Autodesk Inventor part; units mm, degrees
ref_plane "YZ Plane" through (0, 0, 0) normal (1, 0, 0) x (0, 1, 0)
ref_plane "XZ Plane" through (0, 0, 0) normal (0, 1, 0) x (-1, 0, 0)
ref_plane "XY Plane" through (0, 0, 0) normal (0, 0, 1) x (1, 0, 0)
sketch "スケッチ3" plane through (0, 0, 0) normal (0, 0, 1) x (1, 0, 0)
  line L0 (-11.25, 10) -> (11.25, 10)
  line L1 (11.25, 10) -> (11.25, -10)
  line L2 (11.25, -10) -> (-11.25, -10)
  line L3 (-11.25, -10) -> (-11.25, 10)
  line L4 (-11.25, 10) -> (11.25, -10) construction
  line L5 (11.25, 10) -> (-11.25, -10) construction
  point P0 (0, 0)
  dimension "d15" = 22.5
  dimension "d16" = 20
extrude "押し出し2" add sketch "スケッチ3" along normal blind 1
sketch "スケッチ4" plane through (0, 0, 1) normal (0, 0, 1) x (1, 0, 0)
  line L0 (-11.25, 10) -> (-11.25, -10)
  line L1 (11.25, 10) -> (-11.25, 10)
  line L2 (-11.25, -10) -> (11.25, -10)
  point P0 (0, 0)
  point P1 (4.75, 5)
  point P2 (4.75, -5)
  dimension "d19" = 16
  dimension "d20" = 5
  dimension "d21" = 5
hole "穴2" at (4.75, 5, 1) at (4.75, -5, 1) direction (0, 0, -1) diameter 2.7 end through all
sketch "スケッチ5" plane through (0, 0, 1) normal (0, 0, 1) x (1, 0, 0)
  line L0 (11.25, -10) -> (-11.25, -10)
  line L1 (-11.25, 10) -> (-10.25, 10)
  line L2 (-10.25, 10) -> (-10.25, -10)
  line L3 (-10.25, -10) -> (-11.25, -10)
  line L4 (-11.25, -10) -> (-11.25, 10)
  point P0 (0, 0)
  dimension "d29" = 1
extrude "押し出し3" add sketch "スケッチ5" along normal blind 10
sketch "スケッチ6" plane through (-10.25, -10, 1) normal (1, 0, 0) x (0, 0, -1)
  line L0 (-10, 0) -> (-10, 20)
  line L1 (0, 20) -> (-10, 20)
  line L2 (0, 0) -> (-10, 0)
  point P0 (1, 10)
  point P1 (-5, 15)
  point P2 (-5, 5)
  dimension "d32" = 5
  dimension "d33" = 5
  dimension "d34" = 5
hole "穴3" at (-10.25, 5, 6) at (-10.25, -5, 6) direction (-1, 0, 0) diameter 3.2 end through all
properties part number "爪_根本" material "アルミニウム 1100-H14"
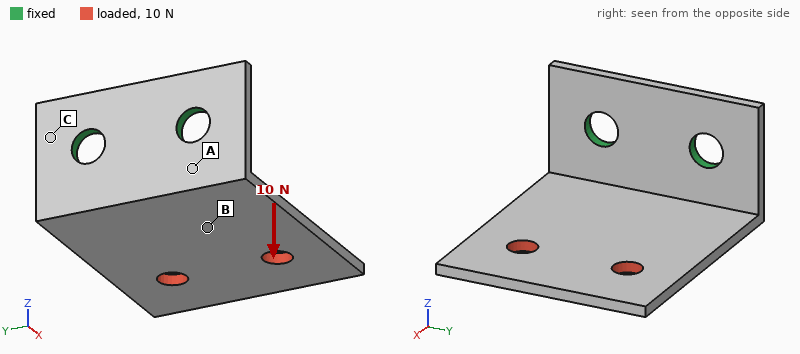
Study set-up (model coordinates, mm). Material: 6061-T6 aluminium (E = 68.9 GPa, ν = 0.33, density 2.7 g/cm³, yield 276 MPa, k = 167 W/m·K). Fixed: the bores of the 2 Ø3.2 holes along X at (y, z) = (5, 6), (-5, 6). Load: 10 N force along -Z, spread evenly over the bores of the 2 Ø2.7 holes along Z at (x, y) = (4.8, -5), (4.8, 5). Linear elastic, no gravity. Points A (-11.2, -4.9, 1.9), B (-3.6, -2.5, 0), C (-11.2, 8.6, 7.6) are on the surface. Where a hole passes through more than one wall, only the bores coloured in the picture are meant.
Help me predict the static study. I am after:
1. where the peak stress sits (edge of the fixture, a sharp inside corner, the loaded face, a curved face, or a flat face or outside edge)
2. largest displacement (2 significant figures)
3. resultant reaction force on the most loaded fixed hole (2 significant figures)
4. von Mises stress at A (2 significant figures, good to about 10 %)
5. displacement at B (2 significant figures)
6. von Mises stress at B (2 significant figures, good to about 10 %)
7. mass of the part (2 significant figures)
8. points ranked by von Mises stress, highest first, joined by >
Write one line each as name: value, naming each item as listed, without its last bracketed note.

where the peak stress sits: a flat face or outside edge
largest displacement: 0.28 mm
resultant reaction force on the most loaded fixed hole: 5.4 N
von Mises stress at A: 42 MPa
displacement at B: 0.068 mm
von Mises stress at B: 22 MPa
mass of the part: 1.7 g
points ranked by von Mises stress, highest first, joined by >: A > B > C
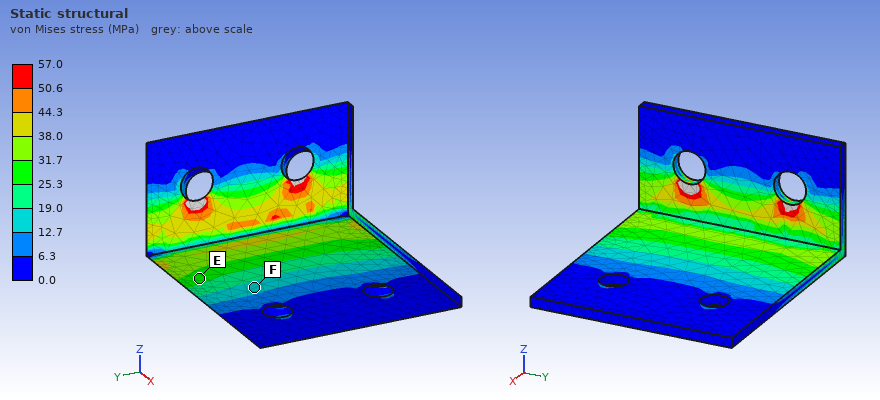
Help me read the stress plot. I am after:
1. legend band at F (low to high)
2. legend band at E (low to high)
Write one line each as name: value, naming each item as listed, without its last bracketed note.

legend band at F: 12.7 to 19.0 MPa
legend band at E: 25.3 to 31.7 MPa
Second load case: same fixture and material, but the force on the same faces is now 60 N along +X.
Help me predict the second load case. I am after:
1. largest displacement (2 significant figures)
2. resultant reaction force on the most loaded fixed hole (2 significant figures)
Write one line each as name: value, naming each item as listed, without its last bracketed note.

largest displacement: 0.11 mm
resultant reaction force on the most loaded fixed hole: 30 N
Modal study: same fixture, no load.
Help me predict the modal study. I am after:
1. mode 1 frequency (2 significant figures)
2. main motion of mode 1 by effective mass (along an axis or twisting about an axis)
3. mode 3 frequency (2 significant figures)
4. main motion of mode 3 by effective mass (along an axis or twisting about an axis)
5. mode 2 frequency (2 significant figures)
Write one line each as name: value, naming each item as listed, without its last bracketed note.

mode 1 frequency: 1300 Hz
main motion of mode 1 by effective mass: along Z
mode 3 frequency: 5300 Hz
main motion of mode 3 by effective mass: along Y
mode 2 frequency: 3700 Hz
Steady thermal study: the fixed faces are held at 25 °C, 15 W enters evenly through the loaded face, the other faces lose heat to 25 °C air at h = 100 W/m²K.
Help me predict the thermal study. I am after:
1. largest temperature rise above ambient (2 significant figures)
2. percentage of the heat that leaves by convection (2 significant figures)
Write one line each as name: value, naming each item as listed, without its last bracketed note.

largest temperature rise above ambient: 75 K
percentage of the heat that leaves by convection: 31 %
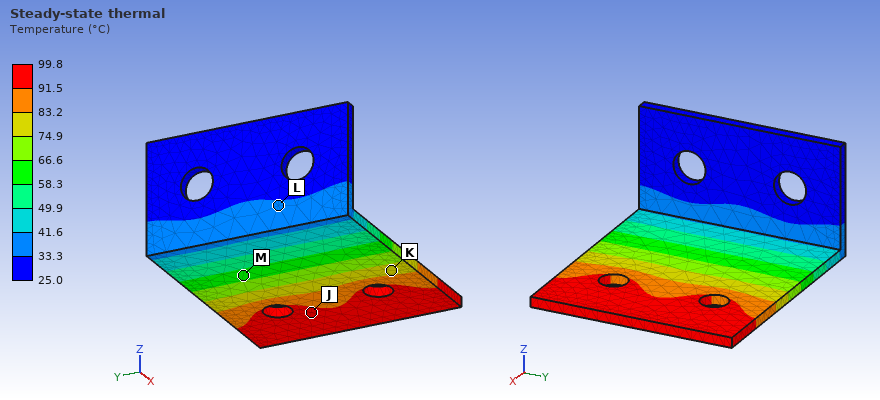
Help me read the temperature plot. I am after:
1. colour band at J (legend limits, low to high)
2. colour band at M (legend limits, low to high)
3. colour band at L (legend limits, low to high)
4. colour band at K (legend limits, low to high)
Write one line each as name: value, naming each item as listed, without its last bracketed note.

colour band at J: 91.5 to 99.8 °C
colour band at M: 58.3 to 66.6 °C
colour band at L: 33.3 to 41.6 °C
colour band at K: 74.9 to 83.2 °C
